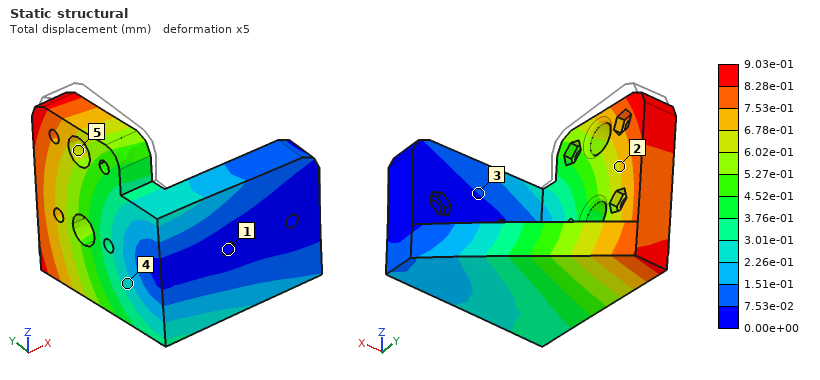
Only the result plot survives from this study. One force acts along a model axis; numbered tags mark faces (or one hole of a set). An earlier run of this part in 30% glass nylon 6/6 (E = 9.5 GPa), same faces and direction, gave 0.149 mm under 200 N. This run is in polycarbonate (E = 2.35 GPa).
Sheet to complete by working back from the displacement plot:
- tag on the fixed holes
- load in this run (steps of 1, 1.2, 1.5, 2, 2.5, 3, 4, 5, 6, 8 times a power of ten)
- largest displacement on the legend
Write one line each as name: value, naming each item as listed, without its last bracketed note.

tag on the fixed holes: 1
load in this run: 300 N
largest displacement on the legend: 9.03e-01 mm
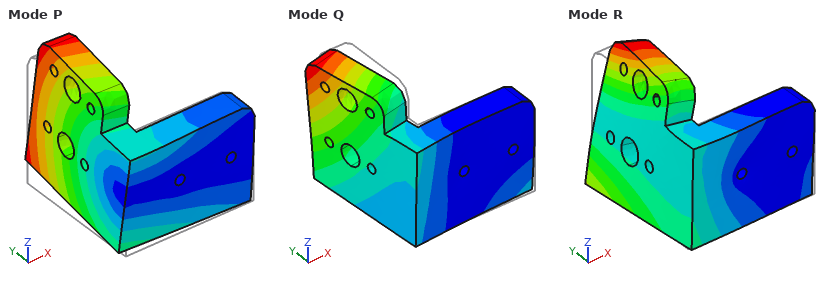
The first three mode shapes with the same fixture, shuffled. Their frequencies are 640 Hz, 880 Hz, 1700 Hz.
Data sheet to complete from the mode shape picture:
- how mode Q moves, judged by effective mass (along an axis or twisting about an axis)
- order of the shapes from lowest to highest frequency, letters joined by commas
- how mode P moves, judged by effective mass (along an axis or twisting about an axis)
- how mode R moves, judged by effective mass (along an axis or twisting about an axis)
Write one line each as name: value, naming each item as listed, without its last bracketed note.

how mode Q moves, judged by effective mass: along X
order of the shapes from lowest to highest frequency, letters joined by commas: P, Q, R
how mode P moves, judged by effective mass: along Z
how mode R moves, judged by effective mass: along Y
